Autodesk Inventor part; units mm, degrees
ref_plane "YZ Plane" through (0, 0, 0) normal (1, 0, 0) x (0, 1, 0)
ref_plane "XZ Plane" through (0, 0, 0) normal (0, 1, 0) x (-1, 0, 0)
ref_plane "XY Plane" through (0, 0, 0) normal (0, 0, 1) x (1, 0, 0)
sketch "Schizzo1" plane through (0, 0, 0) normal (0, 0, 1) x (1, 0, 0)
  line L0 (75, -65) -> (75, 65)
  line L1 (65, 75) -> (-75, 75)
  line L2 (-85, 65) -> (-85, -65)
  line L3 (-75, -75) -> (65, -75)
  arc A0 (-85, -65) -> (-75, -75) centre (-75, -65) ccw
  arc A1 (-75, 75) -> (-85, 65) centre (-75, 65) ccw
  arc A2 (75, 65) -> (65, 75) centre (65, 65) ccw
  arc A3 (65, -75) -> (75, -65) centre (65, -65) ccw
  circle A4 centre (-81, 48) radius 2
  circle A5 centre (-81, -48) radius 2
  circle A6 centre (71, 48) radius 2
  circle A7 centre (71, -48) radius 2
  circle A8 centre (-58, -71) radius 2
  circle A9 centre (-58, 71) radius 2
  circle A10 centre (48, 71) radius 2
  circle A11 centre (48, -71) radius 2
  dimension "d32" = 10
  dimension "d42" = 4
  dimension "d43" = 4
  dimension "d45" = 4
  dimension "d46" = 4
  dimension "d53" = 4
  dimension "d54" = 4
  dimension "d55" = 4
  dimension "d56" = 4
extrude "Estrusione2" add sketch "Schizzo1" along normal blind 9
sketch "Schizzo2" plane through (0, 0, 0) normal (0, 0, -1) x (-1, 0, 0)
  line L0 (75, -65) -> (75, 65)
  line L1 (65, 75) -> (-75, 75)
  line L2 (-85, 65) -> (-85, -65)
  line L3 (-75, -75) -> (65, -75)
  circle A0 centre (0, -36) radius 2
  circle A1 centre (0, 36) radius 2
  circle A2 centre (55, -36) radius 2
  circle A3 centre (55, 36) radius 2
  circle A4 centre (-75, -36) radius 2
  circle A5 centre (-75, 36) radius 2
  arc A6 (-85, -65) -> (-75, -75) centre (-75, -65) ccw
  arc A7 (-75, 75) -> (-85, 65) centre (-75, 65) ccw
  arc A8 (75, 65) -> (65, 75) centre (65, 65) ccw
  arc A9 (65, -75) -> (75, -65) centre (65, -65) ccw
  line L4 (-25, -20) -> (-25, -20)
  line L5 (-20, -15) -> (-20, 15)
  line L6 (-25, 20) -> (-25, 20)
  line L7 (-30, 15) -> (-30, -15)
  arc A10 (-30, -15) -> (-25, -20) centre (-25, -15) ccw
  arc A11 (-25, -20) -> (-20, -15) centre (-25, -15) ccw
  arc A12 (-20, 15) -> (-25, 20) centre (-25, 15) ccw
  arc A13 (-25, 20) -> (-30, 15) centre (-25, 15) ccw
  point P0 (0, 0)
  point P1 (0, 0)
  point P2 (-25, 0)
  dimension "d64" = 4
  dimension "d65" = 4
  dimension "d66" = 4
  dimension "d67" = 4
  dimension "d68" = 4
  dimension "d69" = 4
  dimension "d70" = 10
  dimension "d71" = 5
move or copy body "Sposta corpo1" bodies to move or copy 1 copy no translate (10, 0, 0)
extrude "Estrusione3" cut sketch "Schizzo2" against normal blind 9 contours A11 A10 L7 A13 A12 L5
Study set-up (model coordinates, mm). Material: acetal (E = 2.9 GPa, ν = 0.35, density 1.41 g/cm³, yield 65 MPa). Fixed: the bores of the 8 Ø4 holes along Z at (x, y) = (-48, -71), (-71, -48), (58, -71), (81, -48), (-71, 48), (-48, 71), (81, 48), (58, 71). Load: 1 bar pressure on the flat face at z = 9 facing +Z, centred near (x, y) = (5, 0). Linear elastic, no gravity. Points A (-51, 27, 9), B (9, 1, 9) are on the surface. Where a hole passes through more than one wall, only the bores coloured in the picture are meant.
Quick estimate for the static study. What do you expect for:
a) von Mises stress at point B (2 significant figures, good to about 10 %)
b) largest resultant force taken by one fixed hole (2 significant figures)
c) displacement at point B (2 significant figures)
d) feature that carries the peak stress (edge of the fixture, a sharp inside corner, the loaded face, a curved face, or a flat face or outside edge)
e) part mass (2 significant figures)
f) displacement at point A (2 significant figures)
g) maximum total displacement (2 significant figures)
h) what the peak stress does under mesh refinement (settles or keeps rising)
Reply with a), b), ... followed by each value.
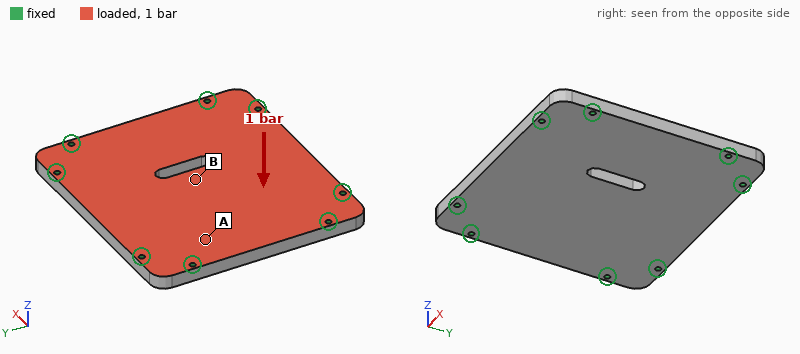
a) 6.4 MPa
b) 320 N
c) 1.0 mm
d) edge of the fixture
e) 300 g
f) 0.38 mm
g) 1.1 mm
h) keeps rising
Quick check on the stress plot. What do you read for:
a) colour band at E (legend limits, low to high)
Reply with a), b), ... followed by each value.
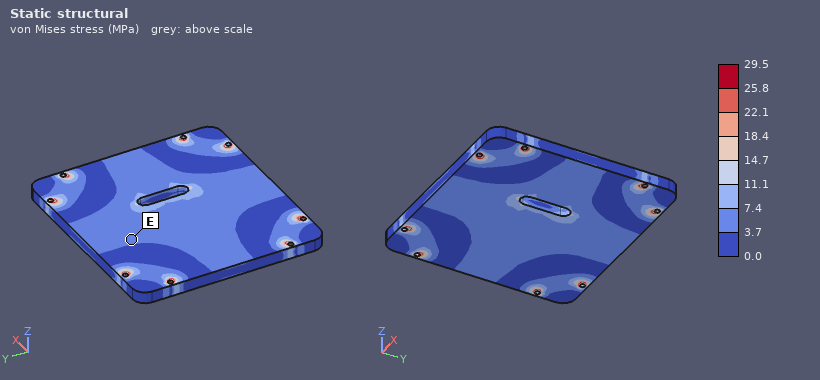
a) 3.7 to 7.4 MPa
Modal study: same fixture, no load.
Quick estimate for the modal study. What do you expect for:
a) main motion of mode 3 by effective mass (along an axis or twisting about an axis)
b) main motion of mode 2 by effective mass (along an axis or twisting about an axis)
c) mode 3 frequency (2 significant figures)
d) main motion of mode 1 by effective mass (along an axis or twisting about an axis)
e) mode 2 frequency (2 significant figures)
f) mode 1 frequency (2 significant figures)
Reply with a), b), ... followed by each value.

a) twisting about Y
b) twisting about X
c) 1100 Hz
d) along Z
e) 1000 Hz
f) 550 Hz
